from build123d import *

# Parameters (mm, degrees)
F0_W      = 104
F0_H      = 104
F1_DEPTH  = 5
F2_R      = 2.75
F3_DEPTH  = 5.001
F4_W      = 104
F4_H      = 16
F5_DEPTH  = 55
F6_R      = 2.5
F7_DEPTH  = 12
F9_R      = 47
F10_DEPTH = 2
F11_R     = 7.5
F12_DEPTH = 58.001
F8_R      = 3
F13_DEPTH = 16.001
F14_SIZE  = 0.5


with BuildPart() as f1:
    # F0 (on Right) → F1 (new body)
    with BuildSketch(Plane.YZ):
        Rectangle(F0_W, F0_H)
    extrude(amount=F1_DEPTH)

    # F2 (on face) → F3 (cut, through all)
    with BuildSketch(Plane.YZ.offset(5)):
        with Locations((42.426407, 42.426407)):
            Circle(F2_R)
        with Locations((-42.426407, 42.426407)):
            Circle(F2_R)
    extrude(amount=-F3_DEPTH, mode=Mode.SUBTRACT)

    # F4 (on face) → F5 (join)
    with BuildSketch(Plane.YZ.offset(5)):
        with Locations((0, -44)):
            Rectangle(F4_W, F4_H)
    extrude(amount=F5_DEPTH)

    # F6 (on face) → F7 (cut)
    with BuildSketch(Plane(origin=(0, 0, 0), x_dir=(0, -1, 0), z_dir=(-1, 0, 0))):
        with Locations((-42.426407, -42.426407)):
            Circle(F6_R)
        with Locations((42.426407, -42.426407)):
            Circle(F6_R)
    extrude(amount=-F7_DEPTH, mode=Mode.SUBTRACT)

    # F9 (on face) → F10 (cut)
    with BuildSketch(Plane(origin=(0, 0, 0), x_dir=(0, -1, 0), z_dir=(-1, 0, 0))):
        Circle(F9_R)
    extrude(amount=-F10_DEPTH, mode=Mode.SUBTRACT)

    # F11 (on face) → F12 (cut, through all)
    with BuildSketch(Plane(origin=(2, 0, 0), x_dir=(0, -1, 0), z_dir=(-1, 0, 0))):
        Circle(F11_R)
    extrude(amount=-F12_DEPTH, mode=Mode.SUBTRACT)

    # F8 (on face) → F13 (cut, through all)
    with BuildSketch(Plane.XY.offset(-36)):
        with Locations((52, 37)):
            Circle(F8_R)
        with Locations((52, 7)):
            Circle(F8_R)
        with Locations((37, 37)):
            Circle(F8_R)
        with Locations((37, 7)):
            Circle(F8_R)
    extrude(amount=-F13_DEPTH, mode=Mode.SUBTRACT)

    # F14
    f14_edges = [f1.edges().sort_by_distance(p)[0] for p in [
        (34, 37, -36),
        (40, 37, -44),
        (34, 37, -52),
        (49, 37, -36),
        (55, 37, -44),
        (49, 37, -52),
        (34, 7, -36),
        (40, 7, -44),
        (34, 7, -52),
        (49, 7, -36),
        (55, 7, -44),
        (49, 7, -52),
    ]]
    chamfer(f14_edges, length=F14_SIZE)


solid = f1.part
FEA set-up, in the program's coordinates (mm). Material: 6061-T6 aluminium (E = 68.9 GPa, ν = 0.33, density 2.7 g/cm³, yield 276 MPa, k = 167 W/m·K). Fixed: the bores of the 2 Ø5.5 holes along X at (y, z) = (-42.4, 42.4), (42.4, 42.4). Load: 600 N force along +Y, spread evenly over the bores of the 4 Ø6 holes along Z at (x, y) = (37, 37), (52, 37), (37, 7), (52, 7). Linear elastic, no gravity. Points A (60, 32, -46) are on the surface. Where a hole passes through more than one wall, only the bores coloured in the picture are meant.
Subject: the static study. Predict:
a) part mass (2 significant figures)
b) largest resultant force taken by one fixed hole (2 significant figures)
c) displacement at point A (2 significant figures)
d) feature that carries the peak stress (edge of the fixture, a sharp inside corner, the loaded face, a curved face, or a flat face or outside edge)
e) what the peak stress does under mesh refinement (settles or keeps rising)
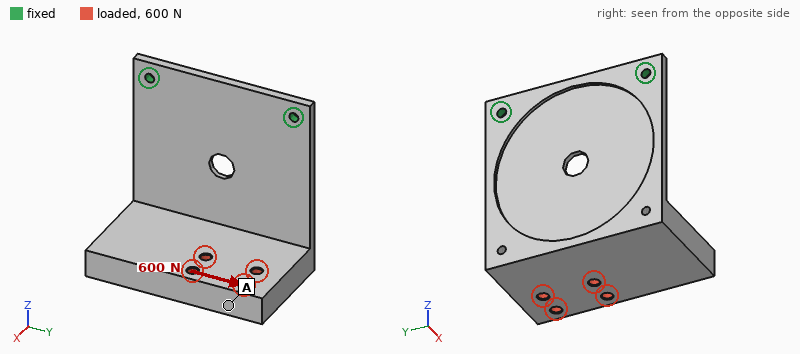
350 g
720 N
0.95 mm
edge of the fixture
keeps rising
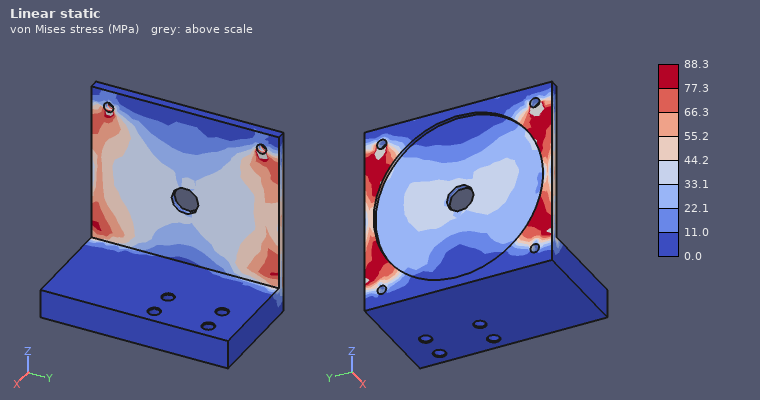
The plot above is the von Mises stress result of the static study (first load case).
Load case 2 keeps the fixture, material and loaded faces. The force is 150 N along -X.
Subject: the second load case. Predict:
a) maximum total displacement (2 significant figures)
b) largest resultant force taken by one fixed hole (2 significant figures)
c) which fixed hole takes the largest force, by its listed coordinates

1.7 mm
220 N
(42.4, 42.4)
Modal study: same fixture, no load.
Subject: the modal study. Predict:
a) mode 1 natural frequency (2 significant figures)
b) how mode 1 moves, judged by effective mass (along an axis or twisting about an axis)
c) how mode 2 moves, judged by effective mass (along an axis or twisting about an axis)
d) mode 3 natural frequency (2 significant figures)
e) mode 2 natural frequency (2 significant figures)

100 Hz
along X
along Y
480 Hz
280 Hz
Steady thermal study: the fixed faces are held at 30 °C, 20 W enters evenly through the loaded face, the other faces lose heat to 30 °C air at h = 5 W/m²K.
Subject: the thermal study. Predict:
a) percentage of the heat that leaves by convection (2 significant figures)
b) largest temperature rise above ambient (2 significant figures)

19 %
31 K
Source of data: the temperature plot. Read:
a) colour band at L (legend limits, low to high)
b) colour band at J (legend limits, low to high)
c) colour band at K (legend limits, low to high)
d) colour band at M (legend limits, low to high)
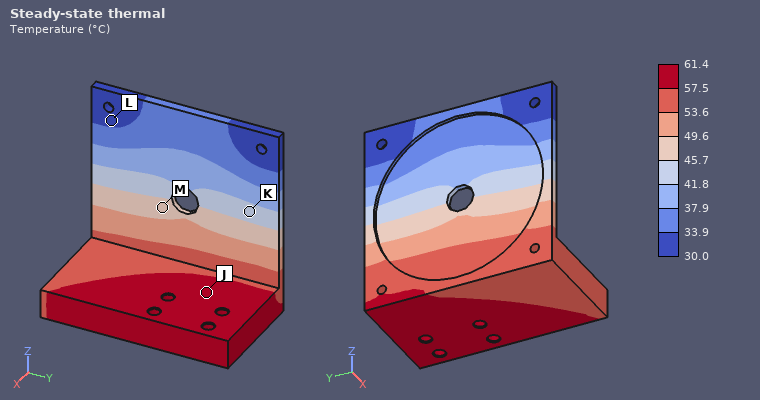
30.0 to 33.9 °C
57.5 to 61.4 °C
41.8 to 45.7 °C
45.7 to 49.6 °C
